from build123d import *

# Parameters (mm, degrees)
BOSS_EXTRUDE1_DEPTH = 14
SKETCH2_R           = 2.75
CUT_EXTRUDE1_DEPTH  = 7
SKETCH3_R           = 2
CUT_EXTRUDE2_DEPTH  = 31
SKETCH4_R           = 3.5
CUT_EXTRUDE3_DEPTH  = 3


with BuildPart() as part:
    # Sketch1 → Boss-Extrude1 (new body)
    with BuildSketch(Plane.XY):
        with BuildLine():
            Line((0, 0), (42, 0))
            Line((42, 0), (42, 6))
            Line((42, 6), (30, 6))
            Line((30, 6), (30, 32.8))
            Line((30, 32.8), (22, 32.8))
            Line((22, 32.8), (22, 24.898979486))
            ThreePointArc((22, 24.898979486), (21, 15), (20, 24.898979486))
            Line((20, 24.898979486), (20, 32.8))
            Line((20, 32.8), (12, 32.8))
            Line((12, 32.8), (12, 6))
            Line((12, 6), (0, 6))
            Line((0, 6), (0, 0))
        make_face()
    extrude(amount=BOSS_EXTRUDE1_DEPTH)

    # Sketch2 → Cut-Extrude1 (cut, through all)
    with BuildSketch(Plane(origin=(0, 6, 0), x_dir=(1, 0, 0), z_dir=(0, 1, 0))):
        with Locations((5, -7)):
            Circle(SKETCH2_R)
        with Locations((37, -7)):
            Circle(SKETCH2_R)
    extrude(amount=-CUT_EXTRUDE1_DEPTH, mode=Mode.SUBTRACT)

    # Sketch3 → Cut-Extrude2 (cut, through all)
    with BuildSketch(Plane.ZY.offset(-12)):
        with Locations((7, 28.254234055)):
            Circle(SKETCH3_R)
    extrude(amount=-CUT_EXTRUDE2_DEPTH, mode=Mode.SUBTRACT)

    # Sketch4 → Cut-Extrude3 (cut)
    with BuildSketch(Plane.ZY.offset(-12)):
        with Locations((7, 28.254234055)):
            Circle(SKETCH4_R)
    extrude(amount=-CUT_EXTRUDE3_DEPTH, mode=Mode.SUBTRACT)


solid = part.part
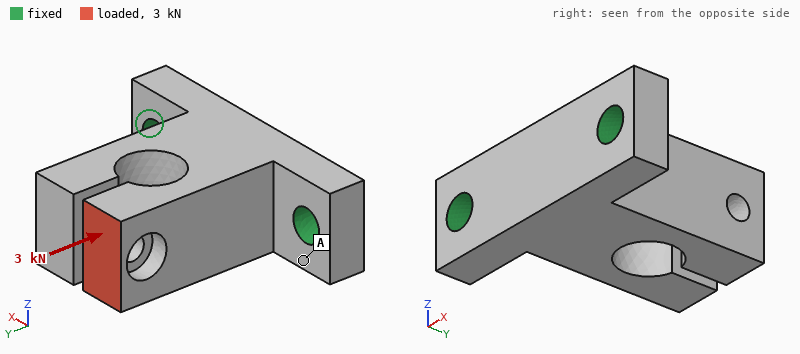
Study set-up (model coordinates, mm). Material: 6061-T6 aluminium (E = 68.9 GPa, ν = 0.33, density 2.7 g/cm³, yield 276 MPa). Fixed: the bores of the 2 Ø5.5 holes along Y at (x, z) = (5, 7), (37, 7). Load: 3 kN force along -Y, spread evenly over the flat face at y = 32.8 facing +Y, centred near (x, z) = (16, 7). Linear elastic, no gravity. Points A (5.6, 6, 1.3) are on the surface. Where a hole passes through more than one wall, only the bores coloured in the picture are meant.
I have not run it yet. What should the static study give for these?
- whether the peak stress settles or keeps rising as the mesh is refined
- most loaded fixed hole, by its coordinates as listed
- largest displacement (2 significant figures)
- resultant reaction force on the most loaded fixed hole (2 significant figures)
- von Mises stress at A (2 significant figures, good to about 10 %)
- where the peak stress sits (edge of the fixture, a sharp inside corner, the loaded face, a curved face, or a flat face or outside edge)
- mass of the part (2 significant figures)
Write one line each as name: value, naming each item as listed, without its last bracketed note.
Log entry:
whether the peak stress settles or keeps rising as the mesh is refined: keeps rising
most loaded fixed hole, by its coordinates as listed: (5, 7)
largest displacement: 0.11 mm
resultant reaction force on the most loaded fixed hole: 2.2 kN
von Mises stress at A: 26 MPa
where the peak stress sits: edge of the fixture
mass of the part: 23 g
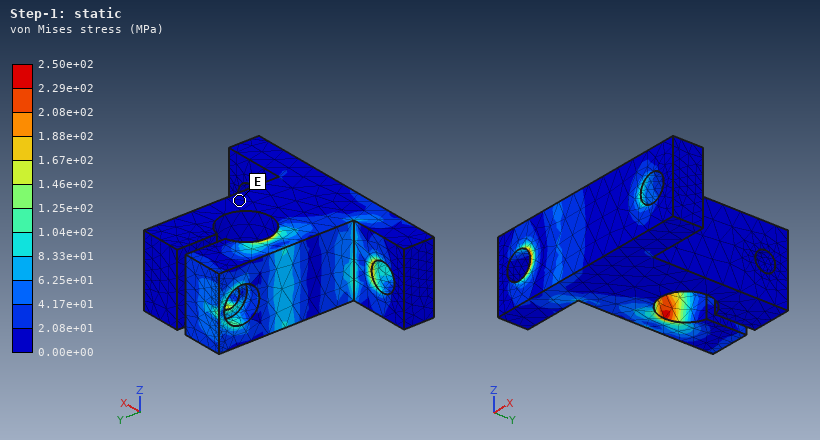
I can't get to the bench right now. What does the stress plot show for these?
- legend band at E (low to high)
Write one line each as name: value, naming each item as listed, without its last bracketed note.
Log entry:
legend band at E: 0.00e+00 to 2.08e+01 MPa
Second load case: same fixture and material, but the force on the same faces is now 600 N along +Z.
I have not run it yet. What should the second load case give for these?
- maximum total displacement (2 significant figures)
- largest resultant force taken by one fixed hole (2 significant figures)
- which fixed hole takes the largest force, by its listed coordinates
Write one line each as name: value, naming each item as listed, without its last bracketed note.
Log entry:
maximum total displacement: 0.15 mm
largest resultant force taken by one fixed hole: 390 N
which fixed hole takes the largest force, by its listed coordinates: (5, 7)
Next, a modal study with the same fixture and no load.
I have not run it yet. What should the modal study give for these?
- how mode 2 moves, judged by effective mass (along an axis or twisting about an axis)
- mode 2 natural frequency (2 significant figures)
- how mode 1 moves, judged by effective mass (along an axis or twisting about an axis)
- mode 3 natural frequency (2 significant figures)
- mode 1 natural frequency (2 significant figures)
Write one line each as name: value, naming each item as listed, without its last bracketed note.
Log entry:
how mode 2 moves, judged by effective mass: along X
mode 2 natural frequency: 7100 Hz
how mode 1 moves, judged by effective mass: along Z
mode 3 natural frequency: 7900 Hz
mode 1 natural frequency: 5300 Hz
